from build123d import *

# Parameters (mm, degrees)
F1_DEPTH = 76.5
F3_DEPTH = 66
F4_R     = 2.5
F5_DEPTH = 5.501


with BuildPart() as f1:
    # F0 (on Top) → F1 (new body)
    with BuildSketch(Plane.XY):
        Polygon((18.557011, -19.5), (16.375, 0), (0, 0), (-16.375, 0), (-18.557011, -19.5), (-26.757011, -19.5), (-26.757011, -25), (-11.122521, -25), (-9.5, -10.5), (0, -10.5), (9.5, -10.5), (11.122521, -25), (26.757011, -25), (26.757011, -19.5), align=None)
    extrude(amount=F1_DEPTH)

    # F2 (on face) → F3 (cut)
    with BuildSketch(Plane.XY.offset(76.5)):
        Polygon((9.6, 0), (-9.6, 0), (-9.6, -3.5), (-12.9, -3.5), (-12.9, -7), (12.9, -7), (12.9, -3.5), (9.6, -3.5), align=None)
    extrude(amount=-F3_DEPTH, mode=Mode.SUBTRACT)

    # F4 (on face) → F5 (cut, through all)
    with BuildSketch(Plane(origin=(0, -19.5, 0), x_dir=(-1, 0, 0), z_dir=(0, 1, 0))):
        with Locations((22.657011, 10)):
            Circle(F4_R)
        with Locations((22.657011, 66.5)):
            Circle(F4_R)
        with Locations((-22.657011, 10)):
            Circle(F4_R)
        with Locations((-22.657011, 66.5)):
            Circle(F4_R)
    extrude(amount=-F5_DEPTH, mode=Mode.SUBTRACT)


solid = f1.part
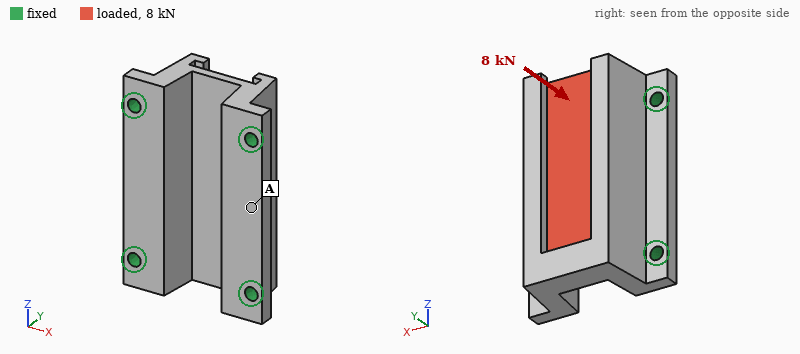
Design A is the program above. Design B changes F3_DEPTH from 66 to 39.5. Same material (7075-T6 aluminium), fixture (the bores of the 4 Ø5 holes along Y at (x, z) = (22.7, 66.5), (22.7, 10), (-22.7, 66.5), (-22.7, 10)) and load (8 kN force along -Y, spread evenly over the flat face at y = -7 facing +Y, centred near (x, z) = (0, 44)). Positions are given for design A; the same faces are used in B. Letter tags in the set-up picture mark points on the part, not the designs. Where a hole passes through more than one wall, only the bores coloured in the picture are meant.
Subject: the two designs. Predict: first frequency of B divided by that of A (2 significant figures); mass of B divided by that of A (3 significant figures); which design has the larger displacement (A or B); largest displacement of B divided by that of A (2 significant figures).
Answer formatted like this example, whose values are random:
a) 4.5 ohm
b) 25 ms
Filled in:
a) 1.1
b) 1.10
c) B
d) 1.3
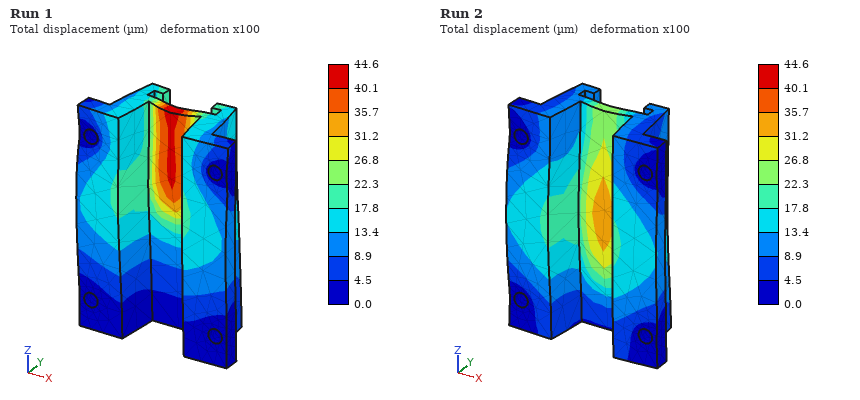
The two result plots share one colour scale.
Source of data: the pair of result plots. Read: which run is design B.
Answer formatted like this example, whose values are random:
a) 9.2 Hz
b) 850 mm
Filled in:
a) Run 1
